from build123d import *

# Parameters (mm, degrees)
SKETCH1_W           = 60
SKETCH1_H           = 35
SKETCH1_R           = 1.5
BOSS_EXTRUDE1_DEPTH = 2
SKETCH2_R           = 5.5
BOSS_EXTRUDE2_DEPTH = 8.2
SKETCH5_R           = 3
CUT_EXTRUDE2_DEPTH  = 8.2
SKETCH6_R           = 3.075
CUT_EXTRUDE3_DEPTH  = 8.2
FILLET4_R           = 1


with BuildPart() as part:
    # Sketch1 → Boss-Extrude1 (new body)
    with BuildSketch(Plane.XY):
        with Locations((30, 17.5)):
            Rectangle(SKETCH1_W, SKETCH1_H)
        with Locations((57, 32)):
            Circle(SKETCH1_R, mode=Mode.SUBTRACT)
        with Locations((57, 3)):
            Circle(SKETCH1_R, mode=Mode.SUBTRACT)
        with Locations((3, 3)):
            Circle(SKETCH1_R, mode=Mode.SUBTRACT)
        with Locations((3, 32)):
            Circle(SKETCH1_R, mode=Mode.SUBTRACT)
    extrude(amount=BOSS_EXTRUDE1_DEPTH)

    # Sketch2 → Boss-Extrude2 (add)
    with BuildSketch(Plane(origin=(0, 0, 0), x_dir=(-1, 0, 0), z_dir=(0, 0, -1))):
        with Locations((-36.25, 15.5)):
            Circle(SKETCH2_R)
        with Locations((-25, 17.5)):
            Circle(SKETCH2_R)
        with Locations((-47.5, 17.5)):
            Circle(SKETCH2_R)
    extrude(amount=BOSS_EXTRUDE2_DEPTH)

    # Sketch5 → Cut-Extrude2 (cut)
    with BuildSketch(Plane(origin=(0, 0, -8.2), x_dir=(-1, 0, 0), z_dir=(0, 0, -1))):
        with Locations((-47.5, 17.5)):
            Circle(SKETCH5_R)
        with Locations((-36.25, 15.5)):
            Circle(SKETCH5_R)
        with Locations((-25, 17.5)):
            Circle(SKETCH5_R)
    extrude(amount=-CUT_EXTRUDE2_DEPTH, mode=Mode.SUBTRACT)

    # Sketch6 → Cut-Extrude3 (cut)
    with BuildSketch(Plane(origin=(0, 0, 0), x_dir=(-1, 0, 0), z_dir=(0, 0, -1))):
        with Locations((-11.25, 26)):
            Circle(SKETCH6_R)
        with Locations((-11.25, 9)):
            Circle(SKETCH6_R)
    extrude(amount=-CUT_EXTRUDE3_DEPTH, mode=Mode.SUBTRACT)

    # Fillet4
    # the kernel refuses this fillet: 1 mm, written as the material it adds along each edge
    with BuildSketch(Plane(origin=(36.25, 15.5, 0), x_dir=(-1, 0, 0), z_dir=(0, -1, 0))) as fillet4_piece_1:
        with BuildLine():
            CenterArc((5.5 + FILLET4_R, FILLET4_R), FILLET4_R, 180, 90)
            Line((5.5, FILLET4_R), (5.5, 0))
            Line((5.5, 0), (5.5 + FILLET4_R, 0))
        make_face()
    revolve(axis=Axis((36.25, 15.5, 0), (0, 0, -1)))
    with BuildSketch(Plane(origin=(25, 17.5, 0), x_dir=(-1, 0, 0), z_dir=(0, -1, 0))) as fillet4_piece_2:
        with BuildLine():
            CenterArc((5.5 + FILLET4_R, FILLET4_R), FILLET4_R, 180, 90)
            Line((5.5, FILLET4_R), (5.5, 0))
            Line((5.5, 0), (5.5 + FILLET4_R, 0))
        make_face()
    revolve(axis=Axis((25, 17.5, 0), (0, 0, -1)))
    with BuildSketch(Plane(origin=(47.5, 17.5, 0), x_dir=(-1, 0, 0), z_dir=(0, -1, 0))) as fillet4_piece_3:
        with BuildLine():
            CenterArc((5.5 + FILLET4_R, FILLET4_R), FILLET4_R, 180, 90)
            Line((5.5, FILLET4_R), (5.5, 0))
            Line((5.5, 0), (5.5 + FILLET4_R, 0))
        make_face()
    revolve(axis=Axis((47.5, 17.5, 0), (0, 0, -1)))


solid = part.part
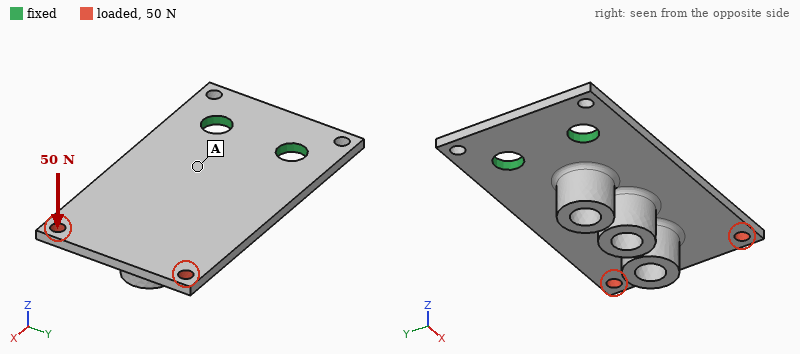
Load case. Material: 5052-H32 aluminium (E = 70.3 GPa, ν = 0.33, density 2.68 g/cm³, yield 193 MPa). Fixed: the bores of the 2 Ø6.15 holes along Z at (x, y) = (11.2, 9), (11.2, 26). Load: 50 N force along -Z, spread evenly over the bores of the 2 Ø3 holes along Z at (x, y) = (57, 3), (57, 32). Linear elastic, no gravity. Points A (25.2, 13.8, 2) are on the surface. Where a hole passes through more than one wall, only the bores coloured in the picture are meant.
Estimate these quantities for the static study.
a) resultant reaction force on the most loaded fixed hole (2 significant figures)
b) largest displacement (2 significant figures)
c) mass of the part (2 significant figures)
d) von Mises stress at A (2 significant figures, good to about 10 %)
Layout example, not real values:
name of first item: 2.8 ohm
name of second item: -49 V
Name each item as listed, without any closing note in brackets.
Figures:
resultant reaction force on the most loaded fixed hole: 31 N
largest displacement: 0.63 mm
mass of the part: 15 g
von Mises stress at A: 19 MPa
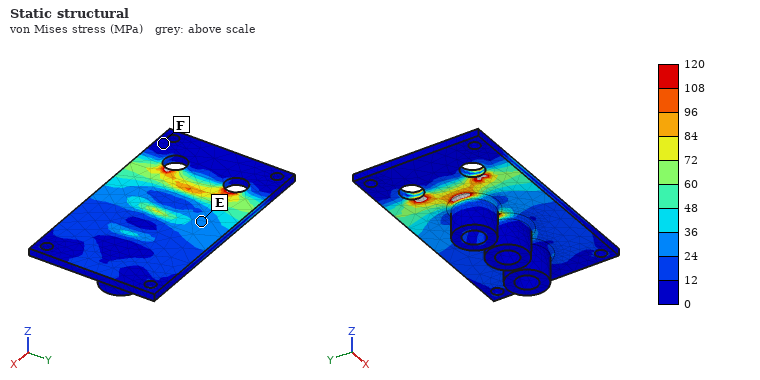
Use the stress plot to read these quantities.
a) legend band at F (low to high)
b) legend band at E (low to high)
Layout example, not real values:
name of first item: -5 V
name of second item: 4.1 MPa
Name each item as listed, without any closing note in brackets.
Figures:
legend band at F: 0 to 12 MPa
legend band at E: 24 to 36 MPa
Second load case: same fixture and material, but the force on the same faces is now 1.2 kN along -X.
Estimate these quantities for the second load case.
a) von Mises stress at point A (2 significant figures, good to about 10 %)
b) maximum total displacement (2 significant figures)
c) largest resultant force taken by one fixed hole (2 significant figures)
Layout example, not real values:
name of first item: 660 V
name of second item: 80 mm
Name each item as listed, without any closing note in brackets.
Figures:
von Mises stress at point A: 18 MPa
maximum total displacement: 32 µm
largest resultant force taken by one fixed hole: 610 N
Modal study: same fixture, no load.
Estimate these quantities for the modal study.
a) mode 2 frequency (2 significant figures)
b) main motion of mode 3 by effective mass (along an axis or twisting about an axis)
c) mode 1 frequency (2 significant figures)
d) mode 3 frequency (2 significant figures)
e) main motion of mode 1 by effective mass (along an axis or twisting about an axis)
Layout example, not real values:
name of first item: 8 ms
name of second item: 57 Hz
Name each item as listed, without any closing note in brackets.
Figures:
mode 2 frequency: 3100 Hz
main motion of mode 3 by effective mass: along Z
mode 1 frequency: 770 Hz
mode 3 frequency: 4900 Hz
main motion of mode 1 by effective mass: along Z
